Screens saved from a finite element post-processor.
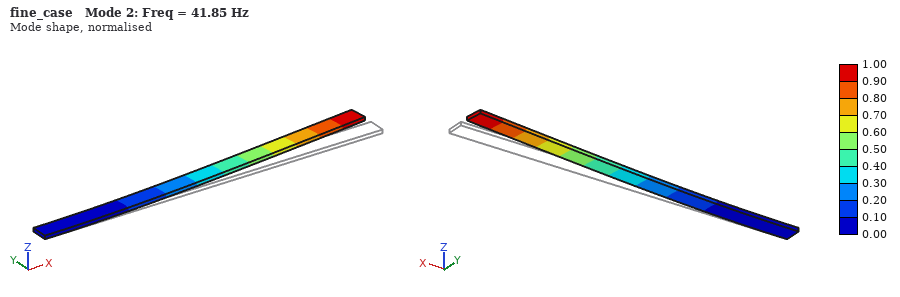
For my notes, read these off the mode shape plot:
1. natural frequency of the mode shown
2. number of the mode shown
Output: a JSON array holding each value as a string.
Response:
["41.85 Hz", "2"]
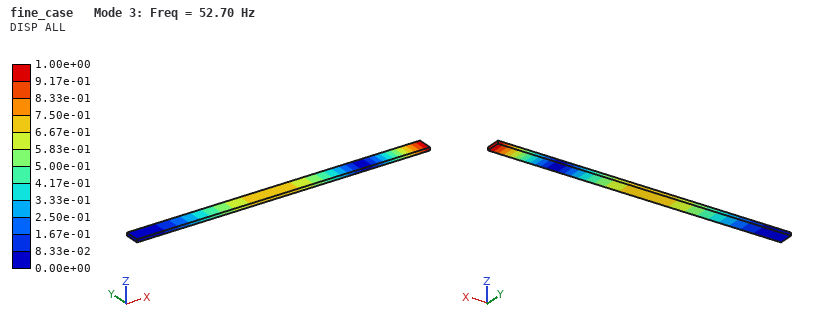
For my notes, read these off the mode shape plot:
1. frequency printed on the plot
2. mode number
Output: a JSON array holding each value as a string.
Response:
["52.70 Hz", "3"]
